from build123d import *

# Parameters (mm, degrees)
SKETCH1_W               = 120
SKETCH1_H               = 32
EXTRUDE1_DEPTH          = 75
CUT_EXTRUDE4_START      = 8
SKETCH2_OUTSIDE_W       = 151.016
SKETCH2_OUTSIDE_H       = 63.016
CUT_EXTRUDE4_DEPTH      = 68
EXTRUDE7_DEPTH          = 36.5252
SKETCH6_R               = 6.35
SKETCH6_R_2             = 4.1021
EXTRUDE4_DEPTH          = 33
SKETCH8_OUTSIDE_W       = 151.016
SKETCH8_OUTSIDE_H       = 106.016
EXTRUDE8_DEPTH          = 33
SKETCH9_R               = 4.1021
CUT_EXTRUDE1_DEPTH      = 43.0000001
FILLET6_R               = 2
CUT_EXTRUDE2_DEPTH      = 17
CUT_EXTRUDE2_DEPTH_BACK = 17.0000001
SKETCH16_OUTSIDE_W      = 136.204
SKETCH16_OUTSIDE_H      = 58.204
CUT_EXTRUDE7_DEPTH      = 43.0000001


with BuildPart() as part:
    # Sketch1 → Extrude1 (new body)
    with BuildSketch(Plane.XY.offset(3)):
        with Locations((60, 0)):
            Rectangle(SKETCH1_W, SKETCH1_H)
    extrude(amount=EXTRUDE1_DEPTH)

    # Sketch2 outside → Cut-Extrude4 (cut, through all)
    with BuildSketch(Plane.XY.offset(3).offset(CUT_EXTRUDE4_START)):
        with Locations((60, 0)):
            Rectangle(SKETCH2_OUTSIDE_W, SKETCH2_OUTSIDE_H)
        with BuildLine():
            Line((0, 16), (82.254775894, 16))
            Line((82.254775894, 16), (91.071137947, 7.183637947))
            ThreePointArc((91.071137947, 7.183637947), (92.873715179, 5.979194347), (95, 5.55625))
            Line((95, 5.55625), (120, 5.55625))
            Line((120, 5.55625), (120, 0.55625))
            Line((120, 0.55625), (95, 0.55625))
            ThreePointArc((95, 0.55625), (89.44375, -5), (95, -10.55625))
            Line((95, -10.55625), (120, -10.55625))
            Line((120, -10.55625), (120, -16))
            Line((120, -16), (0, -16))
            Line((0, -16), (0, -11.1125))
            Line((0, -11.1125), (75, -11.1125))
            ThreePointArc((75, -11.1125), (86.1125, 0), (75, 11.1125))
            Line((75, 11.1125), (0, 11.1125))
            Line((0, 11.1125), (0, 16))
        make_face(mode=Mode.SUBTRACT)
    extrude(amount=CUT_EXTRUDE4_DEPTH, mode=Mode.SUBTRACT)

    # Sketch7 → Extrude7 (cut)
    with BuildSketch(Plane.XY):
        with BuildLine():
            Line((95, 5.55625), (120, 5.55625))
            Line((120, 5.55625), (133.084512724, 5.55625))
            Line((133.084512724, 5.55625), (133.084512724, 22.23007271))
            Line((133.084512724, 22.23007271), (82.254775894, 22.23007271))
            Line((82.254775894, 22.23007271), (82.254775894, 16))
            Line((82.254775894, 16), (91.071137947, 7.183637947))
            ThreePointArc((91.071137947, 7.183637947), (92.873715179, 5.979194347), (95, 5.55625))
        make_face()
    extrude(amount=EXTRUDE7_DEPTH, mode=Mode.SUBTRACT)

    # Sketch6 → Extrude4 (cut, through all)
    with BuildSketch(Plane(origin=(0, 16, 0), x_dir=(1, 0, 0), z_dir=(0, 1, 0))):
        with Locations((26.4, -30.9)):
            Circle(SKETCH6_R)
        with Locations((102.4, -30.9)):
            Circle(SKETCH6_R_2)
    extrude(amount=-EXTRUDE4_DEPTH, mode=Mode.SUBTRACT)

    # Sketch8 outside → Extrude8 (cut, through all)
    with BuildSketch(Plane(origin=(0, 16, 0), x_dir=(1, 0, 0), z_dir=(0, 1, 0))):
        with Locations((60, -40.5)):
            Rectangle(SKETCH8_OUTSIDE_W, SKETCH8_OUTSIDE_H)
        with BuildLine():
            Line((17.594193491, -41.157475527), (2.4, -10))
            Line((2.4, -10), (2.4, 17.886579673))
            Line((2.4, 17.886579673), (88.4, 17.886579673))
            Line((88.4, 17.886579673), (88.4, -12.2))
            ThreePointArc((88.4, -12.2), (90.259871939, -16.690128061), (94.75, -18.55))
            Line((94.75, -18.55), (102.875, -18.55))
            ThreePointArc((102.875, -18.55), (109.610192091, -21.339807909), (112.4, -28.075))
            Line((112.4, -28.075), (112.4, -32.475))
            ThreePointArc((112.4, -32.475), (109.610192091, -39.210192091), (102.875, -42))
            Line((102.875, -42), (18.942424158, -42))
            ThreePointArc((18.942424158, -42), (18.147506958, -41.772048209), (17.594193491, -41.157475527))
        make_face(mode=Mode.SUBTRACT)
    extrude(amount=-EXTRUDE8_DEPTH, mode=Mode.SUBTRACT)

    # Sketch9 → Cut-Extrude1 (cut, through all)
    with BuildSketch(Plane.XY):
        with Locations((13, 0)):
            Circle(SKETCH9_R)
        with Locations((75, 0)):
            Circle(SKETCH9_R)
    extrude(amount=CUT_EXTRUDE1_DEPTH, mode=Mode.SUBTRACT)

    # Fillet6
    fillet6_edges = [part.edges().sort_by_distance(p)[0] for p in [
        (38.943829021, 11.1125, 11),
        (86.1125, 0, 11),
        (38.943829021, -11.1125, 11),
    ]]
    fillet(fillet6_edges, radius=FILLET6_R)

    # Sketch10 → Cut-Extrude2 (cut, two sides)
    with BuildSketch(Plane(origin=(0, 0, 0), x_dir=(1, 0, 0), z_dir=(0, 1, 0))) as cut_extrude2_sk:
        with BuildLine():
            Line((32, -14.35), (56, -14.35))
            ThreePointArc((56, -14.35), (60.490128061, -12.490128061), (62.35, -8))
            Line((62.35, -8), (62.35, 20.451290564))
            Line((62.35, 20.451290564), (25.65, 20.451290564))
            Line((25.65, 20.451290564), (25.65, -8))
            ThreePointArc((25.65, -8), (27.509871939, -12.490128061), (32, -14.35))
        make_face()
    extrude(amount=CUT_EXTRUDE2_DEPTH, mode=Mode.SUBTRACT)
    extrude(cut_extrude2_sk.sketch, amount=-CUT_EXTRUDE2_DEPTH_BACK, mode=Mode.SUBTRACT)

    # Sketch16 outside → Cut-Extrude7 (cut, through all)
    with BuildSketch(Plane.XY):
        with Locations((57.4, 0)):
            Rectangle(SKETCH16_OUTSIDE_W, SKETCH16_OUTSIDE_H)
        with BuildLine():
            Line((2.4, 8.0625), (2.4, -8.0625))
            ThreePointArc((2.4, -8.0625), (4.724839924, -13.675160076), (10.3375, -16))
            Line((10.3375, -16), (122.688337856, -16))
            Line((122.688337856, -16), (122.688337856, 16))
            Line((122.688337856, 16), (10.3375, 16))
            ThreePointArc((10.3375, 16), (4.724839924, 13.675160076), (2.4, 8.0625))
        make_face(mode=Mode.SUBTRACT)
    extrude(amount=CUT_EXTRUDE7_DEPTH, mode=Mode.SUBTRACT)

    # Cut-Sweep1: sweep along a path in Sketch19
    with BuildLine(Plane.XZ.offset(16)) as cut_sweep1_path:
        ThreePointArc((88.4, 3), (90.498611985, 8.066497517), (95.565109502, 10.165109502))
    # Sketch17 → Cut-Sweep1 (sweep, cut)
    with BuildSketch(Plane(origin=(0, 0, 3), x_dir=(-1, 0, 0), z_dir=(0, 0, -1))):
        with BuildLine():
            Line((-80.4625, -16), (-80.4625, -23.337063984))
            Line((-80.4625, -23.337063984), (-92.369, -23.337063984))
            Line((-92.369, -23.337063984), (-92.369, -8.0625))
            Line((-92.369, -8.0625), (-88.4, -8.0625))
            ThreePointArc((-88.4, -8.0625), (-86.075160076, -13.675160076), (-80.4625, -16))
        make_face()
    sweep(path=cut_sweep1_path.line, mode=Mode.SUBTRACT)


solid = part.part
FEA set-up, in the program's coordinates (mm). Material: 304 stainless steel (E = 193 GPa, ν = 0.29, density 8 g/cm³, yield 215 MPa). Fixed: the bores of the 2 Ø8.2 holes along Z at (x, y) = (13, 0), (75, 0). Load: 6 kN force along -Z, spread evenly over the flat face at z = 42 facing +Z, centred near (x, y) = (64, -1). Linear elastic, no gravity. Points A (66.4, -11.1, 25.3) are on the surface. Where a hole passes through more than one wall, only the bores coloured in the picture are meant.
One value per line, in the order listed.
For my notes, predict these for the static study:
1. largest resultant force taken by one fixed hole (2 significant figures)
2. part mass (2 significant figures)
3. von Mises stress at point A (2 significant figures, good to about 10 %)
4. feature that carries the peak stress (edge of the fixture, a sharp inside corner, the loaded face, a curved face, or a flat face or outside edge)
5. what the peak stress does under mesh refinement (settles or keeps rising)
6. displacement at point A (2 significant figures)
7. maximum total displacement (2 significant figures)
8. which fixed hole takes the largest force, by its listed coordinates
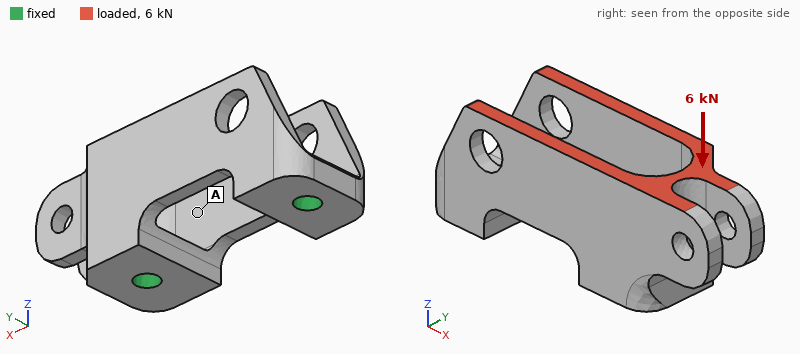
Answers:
4.7 kN
330 g
12 MPa
edge of the fixture
keeps rising
7.3 µm
11 µm
(75, 0)
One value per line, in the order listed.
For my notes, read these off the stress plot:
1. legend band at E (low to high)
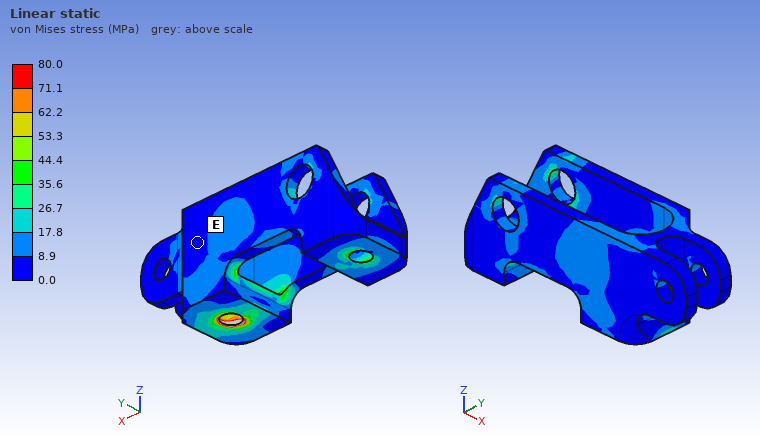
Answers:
0.0 to 8.9 MPa
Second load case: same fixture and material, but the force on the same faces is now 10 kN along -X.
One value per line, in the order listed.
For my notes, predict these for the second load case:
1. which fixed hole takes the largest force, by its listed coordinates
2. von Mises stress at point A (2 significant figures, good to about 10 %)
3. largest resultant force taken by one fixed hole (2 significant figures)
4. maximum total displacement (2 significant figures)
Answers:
(13, 0)
32 MPa
7.3 kN
49 µm
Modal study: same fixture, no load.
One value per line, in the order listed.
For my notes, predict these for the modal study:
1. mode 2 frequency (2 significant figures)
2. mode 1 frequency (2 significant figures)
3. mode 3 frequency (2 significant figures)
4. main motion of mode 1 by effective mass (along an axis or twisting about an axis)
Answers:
3400 Hz
3100 Hz
4700 Hz
along Y
